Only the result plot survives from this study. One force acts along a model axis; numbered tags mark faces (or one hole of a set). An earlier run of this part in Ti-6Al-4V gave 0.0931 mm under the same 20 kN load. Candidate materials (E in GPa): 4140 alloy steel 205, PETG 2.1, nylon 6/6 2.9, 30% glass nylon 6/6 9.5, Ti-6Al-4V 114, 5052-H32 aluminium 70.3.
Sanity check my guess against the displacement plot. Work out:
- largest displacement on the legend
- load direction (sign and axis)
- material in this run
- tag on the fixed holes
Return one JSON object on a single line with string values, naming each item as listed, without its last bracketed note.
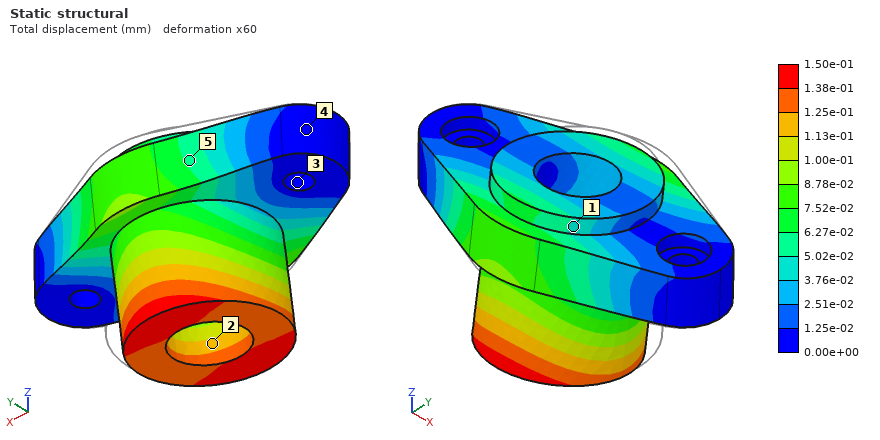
{"largest displacement on the legend": "1.50e-01 mm", "load direction": "-Y", "material in this run": "5052-H32 aluminium", "tag on the fixed holes": "3"}
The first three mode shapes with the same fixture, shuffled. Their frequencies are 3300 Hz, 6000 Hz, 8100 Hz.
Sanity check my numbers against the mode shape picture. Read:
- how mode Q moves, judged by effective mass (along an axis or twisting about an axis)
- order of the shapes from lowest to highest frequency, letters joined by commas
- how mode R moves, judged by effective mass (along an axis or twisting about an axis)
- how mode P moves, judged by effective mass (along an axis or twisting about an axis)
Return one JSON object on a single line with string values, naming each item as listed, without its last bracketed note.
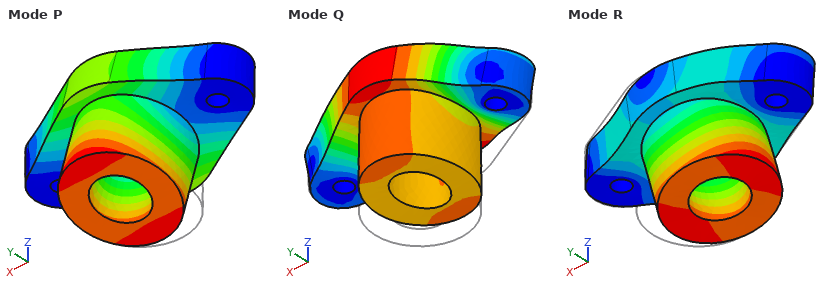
{"how mode Q moves, judged by effective mass": "along Z", "order of the shapes from lowest to highest frequency, letters joined by commas": "P, Q, R", "how mode R moves, judged by effective mass": "along X", "how mode P moves, judged by effective mass": "along Y"}
